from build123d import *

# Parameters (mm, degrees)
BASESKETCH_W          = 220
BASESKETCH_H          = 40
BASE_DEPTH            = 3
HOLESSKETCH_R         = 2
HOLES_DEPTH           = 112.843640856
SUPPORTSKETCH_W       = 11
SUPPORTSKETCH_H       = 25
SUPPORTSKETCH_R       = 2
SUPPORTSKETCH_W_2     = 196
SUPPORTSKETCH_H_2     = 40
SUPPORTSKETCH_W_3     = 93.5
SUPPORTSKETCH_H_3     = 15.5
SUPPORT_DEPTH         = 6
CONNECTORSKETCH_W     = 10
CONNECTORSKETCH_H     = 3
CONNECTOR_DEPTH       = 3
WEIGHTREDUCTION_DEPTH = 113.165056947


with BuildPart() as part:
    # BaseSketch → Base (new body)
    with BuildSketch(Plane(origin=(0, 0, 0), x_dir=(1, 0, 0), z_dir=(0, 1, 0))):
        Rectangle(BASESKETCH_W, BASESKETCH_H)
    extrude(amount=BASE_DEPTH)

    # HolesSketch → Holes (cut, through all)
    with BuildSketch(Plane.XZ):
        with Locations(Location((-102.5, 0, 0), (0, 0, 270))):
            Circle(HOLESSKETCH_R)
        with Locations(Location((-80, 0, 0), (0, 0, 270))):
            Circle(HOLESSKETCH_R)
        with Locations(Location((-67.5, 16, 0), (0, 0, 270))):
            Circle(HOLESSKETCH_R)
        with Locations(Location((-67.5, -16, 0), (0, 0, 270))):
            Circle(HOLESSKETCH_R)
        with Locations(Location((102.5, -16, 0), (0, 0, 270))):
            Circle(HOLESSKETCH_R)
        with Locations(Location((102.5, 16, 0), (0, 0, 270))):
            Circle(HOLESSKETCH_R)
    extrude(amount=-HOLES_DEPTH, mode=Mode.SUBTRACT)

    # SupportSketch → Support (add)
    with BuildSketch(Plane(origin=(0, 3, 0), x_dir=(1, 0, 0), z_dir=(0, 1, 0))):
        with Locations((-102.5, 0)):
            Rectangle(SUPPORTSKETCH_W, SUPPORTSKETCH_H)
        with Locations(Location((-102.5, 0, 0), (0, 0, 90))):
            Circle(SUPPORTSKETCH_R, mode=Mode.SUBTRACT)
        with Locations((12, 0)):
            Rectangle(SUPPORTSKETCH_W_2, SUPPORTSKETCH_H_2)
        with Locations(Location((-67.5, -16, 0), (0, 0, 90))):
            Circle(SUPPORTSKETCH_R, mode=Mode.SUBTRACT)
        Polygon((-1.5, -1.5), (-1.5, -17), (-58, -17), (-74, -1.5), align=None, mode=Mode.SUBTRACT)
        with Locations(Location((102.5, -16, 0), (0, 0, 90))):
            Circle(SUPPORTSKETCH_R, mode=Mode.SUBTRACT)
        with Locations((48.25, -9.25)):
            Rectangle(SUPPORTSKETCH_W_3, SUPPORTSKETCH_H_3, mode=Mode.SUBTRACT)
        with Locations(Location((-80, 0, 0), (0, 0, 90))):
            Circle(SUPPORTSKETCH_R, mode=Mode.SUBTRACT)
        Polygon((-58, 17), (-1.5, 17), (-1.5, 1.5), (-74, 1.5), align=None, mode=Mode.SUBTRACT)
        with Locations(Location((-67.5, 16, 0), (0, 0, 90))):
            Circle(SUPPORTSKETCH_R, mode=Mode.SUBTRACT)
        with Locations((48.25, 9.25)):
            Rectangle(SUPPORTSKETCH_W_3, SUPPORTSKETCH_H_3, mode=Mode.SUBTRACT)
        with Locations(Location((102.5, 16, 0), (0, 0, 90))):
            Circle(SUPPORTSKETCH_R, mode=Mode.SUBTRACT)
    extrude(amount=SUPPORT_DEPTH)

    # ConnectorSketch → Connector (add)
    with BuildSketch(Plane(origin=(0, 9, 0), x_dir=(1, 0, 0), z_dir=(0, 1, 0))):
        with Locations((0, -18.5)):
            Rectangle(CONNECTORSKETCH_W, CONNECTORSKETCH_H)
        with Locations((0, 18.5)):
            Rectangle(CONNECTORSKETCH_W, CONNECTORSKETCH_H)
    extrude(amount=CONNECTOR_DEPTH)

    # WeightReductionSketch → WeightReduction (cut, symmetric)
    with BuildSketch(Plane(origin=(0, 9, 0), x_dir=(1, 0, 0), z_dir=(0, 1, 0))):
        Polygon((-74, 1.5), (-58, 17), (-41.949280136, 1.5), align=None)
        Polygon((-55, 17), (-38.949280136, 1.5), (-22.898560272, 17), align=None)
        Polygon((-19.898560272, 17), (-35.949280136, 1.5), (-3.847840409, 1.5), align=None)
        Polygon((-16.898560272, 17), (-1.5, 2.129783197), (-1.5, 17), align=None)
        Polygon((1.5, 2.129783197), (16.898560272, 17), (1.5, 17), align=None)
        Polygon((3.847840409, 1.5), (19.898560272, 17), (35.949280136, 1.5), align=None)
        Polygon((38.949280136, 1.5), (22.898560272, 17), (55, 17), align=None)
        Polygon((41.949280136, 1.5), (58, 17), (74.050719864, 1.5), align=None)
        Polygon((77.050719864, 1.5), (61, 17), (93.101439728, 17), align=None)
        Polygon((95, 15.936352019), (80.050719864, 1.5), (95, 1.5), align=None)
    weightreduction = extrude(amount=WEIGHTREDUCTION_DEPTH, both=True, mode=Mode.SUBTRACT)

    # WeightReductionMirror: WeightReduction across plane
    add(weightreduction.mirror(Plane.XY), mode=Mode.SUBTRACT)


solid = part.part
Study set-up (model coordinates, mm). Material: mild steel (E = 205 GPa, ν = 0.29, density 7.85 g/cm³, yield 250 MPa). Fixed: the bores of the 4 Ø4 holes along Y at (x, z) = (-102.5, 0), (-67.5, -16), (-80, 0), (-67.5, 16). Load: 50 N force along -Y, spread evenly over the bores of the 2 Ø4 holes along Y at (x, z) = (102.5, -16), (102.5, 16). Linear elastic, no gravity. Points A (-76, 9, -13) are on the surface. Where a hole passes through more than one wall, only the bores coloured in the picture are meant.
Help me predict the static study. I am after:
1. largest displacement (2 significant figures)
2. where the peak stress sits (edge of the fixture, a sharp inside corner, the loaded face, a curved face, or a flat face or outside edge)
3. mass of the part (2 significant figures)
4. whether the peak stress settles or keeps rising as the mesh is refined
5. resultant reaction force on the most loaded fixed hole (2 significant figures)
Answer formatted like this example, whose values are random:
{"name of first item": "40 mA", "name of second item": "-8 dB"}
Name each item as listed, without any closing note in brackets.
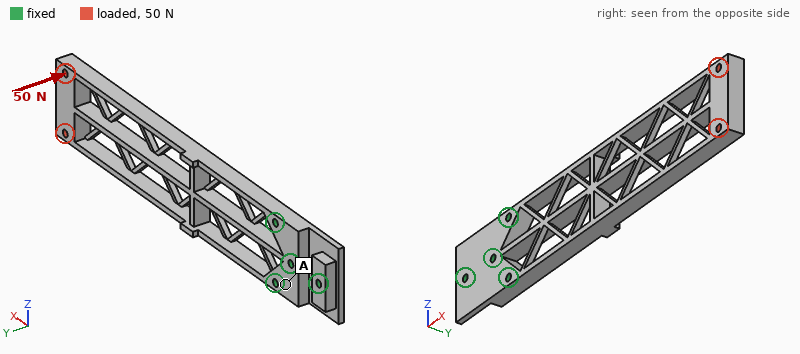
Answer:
{"largest displacement": "0.73 mm", "where the peak stress sits": "a sharp inside corner", "mass of the part": "260 g", "whether the peak stress settles or keeps rising as the mesh is refined": "keeps rising", "resultant reaction force on the most loaded fixed hole": "80 N"}
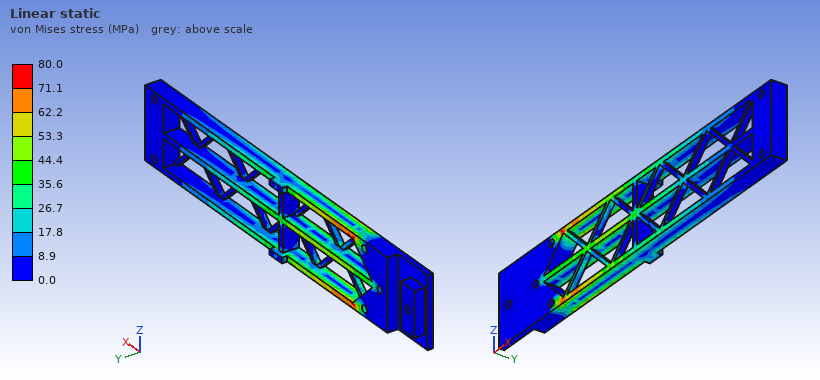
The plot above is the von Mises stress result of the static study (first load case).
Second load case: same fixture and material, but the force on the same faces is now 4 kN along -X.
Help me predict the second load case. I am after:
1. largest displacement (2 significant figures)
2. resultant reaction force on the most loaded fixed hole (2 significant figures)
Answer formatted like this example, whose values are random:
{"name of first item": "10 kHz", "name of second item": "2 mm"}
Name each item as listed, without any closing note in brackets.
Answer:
{"largest displacement": "45 µm", "resultant reaction force on the most loaded fixed hole": "1.5 kN"}
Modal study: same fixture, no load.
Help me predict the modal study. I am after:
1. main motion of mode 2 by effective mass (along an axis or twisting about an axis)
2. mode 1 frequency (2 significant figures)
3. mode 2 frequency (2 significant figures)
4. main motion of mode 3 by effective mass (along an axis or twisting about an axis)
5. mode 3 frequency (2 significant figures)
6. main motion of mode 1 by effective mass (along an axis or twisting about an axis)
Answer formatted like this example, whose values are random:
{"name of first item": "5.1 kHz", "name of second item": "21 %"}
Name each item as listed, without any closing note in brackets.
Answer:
{"main motion of mode 2 by effective mass": "along Z", "mode 1 frequency": "170 Hz", "mode 2 frequency": "550 Hz", "main motion of mode 3 by effective mass": "along Z", "mode 3 frequency": "880 Hz", "main motion of mode 1 by effective mass": "along Y"}
